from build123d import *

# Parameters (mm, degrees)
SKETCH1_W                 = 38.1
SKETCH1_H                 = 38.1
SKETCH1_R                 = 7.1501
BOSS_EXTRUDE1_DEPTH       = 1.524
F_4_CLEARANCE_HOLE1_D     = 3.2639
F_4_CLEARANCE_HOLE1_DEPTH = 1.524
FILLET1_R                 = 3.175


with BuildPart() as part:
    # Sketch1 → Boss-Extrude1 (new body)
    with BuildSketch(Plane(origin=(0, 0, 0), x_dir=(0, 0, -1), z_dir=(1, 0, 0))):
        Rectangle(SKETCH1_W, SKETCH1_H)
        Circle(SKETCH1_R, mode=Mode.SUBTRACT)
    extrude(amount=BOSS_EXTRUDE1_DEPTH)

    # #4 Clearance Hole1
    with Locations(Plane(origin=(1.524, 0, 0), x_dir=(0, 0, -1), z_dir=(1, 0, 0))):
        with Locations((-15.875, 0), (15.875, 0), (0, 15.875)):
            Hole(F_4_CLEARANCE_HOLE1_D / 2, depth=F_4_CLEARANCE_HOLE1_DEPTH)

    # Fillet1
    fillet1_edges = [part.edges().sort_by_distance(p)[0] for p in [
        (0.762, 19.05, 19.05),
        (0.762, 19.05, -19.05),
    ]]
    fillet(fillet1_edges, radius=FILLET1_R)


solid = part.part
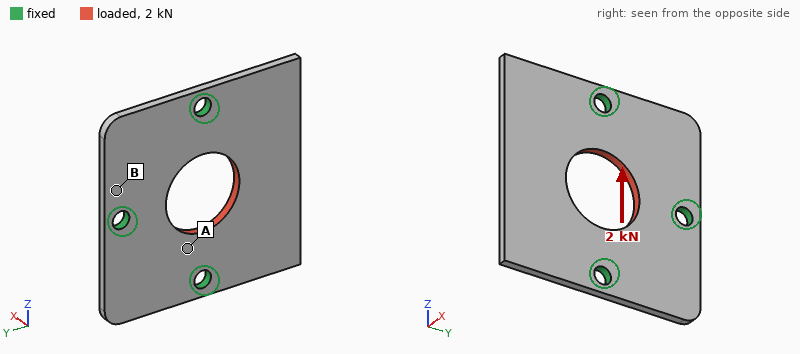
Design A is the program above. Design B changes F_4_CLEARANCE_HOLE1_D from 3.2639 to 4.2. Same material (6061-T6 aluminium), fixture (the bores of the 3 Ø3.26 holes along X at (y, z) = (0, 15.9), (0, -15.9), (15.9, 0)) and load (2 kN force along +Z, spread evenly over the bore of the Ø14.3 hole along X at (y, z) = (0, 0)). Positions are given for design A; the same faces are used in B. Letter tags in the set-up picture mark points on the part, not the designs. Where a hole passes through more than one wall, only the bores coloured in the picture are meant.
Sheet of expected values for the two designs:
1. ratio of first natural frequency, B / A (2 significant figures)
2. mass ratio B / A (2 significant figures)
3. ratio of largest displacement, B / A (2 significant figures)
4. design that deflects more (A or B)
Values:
1.1
0.99
0.92
A
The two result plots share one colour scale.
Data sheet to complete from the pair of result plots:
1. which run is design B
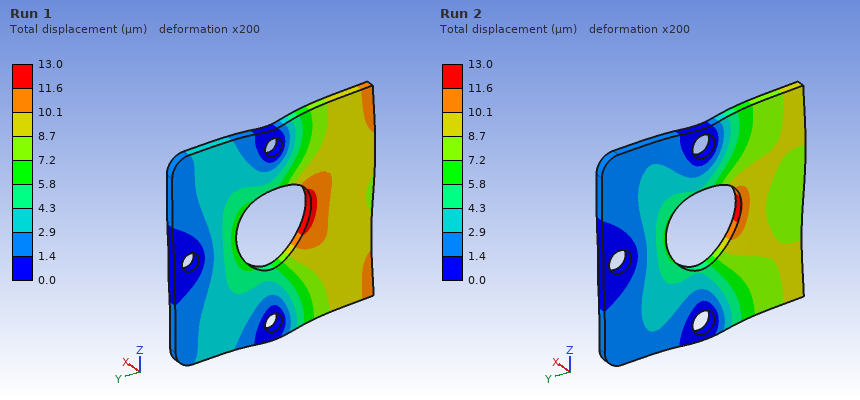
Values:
Run 2
